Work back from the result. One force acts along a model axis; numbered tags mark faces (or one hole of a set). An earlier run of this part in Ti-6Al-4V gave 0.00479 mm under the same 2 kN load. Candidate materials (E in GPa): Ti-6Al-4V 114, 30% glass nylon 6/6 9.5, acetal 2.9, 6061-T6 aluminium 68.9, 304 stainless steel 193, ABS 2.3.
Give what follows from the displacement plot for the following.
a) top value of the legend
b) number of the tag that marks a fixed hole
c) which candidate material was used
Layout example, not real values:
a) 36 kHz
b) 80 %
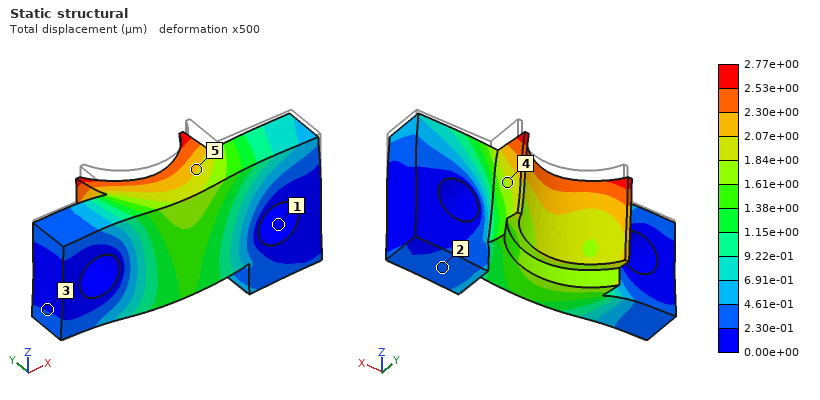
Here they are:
a) 2.77e+00 µm
b) 1
c) 304 stainless steel
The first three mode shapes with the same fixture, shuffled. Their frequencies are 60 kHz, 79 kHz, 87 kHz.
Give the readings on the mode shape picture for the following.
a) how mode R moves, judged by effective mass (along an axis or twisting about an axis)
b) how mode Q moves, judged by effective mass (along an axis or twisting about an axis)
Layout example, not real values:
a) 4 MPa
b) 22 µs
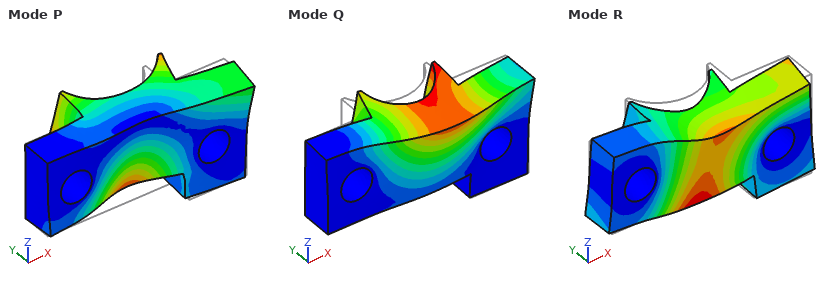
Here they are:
a) along Z
b) along Y
